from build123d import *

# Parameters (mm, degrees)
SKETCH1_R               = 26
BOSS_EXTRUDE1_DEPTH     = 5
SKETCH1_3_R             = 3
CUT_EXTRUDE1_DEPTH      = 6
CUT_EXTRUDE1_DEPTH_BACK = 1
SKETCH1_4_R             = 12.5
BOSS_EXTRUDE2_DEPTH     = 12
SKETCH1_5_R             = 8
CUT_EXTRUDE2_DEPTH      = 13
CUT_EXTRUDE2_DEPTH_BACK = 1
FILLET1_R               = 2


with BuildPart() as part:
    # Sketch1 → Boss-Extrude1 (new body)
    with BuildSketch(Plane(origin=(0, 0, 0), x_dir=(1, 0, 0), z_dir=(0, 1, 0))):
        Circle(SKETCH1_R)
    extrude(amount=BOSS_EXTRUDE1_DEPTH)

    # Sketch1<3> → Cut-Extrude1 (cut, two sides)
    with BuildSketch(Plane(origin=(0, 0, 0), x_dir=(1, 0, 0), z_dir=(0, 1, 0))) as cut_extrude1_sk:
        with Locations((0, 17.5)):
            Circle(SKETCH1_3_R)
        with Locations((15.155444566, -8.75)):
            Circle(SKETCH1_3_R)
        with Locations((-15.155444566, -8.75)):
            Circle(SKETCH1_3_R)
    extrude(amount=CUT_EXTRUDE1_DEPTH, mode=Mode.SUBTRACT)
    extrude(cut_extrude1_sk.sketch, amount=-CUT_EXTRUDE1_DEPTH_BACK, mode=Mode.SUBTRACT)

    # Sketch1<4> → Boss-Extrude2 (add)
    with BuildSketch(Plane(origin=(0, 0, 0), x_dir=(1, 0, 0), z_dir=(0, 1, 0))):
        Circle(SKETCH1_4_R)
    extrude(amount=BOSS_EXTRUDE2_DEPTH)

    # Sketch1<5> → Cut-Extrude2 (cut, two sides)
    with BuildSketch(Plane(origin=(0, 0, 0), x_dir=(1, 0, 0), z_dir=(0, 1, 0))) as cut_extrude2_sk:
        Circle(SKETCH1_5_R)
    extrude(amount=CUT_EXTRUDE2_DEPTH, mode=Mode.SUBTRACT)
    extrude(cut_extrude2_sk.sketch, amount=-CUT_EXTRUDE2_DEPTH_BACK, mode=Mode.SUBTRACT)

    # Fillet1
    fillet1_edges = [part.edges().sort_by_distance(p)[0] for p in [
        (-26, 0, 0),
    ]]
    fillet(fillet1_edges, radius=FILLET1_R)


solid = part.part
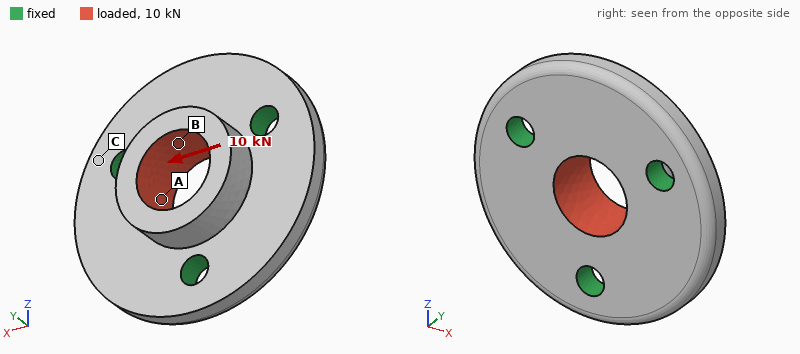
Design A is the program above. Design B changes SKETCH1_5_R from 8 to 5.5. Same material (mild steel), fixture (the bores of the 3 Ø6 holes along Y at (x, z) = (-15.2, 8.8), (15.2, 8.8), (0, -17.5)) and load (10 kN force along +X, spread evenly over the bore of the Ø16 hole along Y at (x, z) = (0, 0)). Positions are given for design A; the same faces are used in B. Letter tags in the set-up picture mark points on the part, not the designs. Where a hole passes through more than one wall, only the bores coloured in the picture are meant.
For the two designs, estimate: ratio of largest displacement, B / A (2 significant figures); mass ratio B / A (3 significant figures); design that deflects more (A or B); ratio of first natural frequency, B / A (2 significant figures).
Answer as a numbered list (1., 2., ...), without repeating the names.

1. 0.77
2. 1.11
3. A
4. 1.0
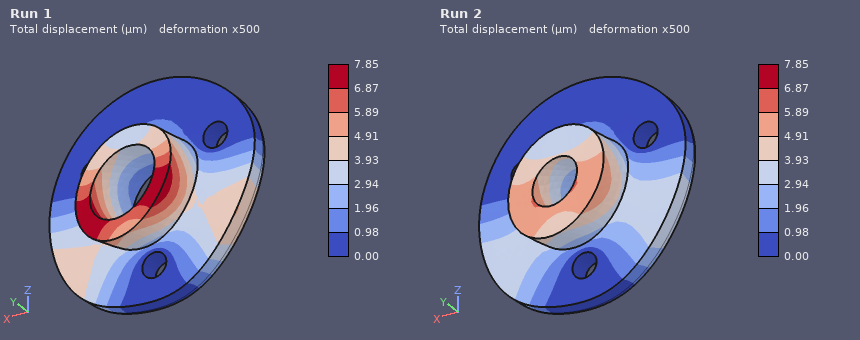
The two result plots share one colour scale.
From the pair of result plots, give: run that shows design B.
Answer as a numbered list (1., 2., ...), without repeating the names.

1. Run 2
